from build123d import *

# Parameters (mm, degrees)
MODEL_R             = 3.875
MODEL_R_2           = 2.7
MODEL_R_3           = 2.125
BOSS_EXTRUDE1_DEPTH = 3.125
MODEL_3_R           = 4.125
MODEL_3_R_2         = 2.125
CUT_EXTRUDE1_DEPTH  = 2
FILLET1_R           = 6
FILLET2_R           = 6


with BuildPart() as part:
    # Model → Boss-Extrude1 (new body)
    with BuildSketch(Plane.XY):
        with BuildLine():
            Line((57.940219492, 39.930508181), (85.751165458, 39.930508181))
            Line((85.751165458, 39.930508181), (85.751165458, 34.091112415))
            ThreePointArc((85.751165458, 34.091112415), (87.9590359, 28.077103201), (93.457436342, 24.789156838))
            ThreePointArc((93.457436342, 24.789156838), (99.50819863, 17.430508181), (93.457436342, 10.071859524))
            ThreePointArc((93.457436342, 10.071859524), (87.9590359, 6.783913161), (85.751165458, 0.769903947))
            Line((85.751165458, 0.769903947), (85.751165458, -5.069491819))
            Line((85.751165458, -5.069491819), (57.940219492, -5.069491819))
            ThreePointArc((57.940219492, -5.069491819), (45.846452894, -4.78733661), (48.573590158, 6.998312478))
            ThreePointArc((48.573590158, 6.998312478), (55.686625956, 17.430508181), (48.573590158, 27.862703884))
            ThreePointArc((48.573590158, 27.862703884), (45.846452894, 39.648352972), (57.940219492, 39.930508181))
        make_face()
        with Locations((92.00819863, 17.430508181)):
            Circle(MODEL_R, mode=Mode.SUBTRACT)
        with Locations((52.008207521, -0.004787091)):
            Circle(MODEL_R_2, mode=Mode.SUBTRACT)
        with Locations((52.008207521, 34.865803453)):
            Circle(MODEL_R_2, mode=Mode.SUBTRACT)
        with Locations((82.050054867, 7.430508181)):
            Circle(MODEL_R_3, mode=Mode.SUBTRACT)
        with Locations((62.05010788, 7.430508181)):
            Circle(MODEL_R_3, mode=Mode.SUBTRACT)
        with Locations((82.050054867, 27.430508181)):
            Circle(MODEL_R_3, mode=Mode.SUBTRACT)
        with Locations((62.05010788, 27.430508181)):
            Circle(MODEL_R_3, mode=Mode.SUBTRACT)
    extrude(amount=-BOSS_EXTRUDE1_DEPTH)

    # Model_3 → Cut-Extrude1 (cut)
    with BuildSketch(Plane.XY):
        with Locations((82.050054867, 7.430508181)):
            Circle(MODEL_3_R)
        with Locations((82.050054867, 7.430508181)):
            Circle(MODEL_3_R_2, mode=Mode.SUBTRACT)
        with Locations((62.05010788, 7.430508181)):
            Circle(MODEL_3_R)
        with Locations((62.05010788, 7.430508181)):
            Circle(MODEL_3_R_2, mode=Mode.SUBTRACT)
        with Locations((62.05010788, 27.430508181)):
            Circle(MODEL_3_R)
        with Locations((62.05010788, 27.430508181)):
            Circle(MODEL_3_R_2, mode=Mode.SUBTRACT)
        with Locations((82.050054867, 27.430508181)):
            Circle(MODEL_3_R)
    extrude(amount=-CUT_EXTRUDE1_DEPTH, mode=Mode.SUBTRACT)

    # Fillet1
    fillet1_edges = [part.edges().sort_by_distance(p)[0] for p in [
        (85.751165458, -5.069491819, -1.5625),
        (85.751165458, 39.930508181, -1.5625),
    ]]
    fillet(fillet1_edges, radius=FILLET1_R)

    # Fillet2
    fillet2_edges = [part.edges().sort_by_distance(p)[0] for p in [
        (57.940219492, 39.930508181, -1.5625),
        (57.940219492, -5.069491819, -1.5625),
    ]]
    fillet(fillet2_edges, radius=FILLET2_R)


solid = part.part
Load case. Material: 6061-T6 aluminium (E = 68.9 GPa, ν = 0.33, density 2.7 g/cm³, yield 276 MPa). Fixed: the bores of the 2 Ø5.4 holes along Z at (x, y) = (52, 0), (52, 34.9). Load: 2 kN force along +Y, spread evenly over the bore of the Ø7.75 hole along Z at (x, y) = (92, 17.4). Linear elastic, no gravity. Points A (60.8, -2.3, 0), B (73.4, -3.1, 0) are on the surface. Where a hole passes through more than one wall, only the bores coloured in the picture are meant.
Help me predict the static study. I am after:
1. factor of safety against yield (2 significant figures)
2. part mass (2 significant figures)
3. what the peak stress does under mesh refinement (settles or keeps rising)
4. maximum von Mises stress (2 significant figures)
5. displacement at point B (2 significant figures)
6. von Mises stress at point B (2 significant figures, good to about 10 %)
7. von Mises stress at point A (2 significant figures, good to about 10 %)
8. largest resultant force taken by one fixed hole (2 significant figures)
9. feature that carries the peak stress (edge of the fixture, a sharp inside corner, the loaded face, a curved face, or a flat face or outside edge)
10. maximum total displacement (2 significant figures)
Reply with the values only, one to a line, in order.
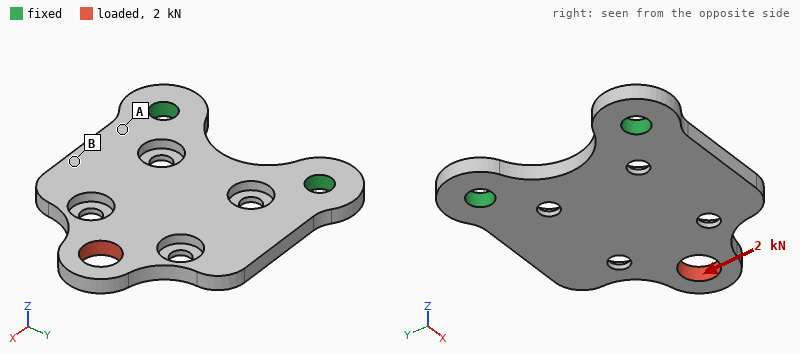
1.1
14 g
settles
250 MPa
0.034 mm
29 MPa
60 MPa
2.3 kN
a curved face
0.10 mm
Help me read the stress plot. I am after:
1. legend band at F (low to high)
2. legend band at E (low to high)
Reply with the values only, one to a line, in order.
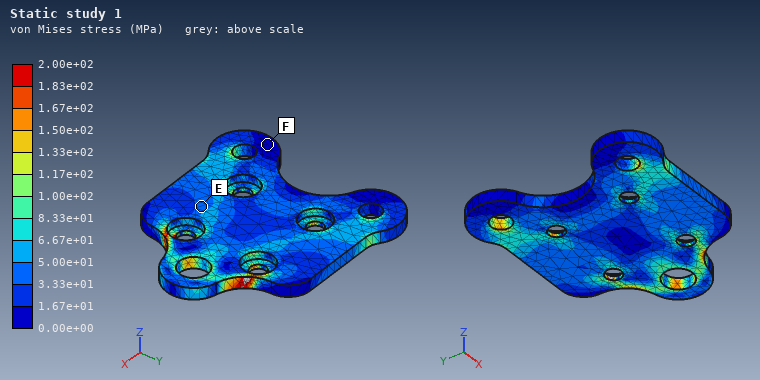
0.00e+00 to 1.67e+01 MPa
3.33e+01 to 5.00e+01 MPa
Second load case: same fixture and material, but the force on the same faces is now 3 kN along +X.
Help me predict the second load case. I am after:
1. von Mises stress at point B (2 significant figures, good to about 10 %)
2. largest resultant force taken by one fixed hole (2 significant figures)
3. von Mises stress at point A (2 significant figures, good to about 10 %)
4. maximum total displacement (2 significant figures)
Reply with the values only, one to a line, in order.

18 MPa
1.6 kN
39 MPa
80 µm
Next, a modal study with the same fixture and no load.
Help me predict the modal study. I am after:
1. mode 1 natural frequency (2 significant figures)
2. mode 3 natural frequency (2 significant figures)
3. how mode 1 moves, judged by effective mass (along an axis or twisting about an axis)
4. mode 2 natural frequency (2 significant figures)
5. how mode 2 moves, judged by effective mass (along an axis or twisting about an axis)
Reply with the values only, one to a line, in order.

1600 Hz
7200 Hz
along Z
4700 Hz
twisting about X
